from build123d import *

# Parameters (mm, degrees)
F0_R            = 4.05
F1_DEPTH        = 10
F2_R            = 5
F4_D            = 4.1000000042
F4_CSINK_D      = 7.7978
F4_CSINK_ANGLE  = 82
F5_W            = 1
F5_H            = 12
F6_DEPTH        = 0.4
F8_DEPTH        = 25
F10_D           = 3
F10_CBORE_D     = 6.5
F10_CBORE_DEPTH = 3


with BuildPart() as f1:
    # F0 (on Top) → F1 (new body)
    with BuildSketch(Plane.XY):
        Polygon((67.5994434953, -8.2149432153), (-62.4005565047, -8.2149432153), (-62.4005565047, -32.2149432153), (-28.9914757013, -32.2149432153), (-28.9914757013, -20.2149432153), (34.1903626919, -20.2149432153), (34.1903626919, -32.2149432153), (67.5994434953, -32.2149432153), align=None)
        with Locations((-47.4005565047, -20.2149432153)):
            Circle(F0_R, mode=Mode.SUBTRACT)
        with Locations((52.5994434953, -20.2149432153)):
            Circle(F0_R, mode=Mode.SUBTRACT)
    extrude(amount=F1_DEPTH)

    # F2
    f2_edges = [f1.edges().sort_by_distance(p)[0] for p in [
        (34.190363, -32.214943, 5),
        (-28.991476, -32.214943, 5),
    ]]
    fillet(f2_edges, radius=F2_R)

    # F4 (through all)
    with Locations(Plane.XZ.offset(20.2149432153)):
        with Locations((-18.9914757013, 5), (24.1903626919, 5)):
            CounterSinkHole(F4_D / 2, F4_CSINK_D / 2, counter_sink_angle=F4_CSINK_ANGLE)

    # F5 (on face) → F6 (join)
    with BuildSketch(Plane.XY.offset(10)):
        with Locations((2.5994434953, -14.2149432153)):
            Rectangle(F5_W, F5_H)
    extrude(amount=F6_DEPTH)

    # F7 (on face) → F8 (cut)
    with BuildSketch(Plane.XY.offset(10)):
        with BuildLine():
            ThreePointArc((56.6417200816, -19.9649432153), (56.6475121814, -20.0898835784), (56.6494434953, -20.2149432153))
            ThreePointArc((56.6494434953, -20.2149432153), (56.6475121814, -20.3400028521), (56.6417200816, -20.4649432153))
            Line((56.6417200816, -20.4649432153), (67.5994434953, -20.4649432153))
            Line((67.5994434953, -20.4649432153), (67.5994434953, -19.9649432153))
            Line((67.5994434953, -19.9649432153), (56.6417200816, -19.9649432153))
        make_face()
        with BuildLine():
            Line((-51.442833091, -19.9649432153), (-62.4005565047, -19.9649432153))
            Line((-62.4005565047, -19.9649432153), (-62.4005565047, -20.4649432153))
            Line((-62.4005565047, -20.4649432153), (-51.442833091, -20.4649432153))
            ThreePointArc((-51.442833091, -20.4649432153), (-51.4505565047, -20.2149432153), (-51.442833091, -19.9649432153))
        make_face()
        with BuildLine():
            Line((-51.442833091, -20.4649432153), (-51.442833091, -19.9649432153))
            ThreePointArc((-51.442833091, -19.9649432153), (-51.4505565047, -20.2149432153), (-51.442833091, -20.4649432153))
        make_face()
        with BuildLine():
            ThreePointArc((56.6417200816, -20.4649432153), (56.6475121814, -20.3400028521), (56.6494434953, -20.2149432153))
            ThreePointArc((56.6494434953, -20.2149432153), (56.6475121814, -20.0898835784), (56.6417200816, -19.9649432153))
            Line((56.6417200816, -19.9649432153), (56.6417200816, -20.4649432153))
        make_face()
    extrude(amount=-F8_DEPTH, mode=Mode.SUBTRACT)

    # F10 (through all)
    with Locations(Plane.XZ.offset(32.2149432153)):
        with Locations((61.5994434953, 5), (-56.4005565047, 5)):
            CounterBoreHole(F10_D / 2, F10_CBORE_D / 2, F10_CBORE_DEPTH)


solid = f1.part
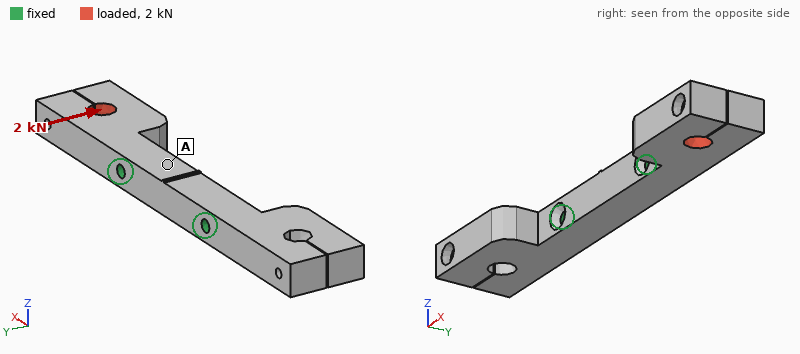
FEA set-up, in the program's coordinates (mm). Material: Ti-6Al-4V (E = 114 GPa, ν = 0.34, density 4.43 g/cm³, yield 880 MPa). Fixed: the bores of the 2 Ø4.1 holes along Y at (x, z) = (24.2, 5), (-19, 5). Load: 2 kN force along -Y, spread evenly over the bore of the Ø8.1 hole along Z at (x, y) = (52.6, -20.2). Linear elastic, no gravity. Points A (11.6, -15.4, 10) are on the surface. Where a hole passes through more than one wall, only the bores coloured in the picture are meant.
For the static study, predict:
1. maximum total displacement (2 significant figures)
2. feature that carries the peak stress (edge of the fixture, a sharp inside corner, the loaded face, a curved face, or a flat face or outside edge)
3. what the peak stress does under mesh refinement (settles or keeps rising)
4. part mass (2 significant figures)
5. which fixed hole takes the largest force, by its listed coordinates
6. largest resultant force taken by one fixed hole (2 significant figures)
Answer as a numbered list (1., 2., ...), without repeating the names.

1. 0.20 mm
2. edge of the fixture
3. keeps rising
4. 95 g
5. (24.2, 5)
6. 2.1 kN
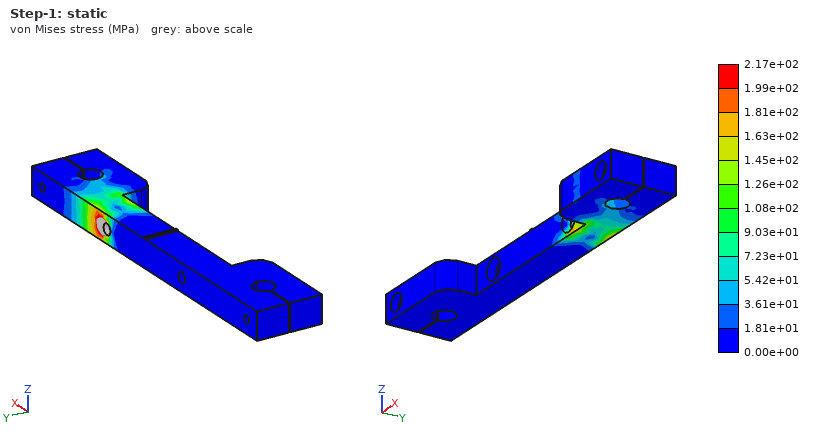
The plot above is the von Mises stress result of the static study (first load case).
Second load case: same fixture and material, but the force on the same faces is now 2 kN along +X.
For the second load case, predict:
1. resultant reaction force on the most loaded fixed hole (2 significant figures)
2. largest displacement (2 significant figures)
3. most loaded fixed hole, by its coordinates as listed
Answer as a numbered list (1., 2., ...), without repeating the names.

1. 1.9 kN
2. 55 µm
3. (24.2, 5)
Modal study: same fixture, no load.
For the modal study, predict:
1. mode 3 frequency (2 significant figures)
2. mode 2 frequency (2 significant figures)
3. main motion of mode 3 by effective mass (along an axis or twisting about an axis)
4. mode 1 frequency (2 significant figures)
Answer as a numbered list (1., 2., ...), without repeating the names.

1. 3600 Hz
2. 2900 Hz
3. along Y
4. 2900 Hz
